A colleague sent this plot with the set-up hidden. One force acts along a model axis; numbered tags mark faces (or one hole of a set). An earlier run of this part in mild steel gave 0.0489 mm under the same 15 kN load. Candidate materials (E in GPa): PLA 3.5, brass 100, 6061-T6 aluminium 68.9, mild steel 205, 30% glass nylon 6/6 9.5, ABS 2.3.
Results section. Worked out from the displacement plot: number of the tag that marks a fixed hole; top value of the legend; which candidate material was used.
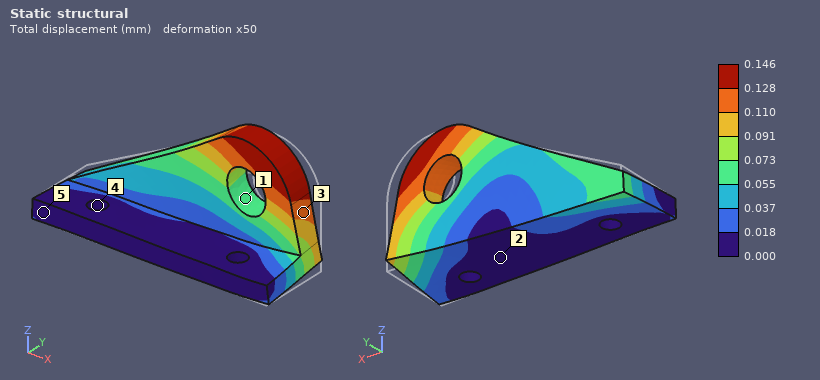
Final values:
4
0.146 mm
6061-T6 aluminium
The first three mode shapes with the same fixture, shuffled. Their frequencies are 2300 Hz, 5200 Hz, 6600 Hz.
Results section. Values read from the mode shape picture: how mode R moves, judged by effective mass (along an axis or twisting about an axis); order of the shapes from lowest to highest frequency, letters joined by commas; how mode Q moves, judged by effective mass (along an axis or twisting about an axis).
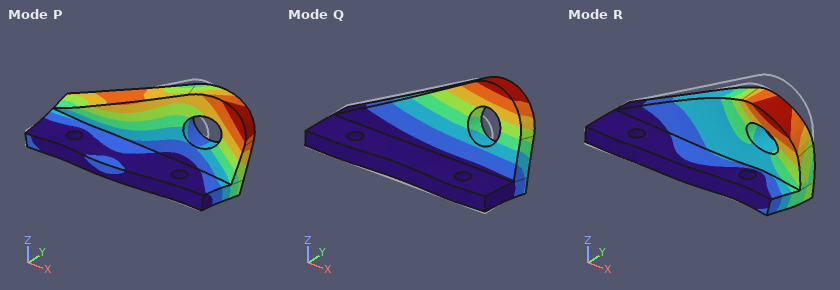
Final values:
along Z
Q, P, R
along Y
